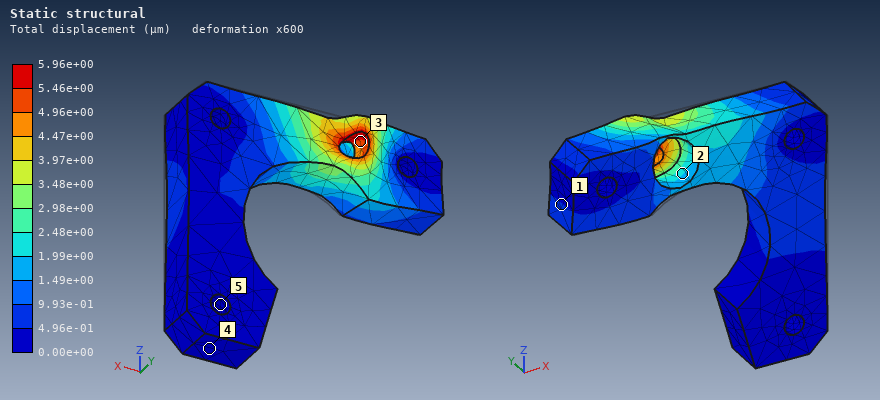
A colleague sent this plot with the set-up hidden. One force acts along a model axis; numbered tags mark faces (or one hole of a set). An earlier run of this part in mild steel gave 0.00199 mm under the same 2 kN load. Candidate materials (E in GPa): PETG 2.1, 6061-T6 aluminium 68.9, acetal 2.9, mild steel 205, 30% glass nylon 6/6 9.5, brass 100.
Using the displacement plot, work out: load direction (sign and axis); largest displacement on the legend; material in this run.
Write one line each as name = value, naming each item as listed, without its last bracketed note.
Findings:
load direction = -X
largest displacement on the legend = 5.96e+00 µm
material in this run = 6061-T6 aluminium
